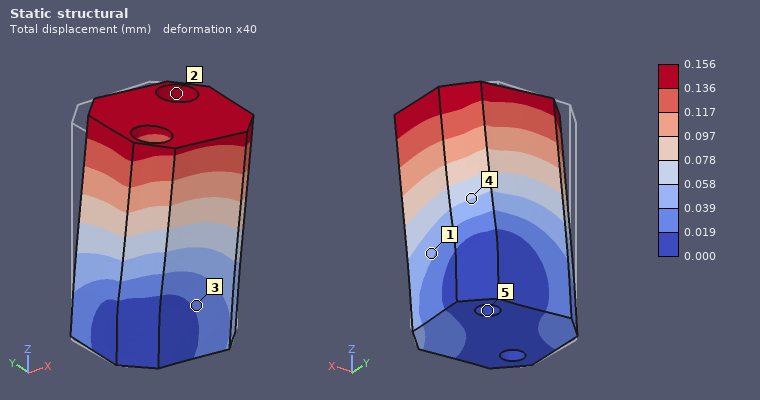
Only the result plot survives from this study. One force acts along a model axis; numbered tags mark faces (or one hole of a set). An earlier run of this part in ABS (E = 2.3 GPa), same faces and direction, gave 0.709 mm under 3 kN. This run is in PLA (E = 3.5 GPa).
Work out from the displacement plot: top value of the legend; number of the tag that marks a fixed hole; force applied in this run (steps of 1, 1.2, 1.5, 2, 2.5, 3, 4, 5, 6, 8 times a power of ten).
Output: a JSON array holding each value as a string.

["0.156 mm", "5", "1 kN"]
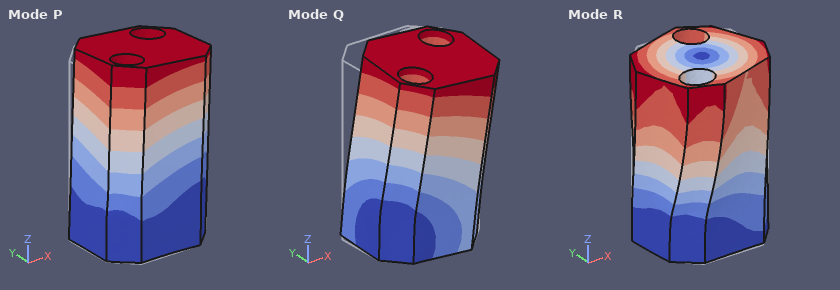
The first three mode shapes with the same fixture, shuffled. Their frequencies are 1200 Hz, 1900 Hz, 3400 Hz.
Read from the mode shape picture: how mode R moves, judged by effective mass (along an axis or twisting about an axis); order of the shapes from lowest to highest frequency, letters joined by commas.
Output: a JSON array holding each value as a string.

["twisting about Z", "Q, P, R"]
